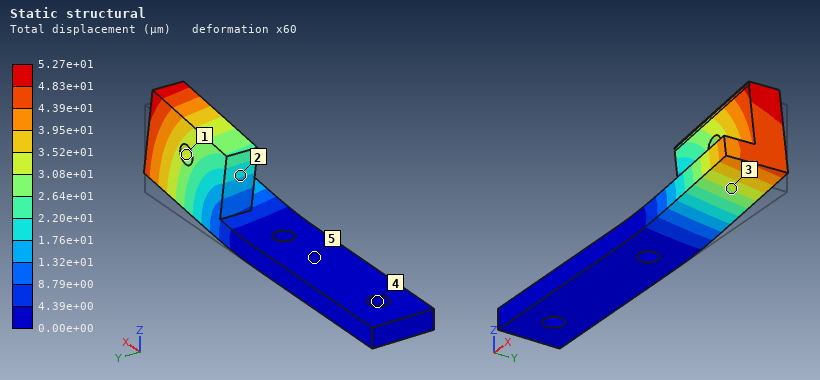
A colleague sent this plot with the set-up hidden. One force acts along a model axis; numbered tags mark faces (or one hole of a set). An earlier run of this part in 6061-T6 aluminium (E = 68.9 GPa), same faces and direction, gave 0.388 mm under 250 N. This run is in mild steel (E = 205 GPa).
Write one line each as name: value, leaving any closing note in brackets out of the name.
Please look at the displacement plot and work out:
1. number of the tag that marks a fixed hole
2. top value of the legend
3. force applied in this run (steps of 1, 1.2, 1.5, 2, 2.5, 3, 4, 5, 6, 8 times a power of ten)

number of the tag that marks a fixed hole: 4
top value of the legend: 5.27e+01 µm
force applied in this run: 100 N
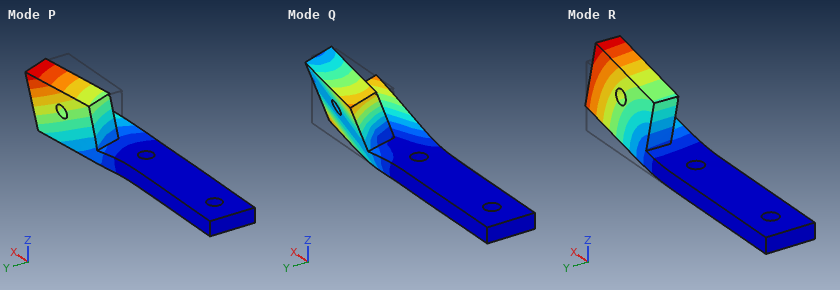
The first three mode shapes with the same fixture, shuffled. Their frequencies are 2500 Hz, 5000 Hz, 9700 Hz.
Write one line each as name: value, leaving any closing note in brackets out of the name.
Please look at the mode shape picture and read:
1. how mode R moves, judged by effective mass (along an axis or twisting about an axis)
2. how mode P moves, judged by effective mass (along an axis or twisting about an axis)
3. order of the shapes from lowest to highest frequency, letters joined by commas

how mode R moves, judged by effective mass: along Z
how mode P moves, judged by effective mass: along Y
order of the shapes from lowest to highest frequency, letters joined by commas: R, P, Q
